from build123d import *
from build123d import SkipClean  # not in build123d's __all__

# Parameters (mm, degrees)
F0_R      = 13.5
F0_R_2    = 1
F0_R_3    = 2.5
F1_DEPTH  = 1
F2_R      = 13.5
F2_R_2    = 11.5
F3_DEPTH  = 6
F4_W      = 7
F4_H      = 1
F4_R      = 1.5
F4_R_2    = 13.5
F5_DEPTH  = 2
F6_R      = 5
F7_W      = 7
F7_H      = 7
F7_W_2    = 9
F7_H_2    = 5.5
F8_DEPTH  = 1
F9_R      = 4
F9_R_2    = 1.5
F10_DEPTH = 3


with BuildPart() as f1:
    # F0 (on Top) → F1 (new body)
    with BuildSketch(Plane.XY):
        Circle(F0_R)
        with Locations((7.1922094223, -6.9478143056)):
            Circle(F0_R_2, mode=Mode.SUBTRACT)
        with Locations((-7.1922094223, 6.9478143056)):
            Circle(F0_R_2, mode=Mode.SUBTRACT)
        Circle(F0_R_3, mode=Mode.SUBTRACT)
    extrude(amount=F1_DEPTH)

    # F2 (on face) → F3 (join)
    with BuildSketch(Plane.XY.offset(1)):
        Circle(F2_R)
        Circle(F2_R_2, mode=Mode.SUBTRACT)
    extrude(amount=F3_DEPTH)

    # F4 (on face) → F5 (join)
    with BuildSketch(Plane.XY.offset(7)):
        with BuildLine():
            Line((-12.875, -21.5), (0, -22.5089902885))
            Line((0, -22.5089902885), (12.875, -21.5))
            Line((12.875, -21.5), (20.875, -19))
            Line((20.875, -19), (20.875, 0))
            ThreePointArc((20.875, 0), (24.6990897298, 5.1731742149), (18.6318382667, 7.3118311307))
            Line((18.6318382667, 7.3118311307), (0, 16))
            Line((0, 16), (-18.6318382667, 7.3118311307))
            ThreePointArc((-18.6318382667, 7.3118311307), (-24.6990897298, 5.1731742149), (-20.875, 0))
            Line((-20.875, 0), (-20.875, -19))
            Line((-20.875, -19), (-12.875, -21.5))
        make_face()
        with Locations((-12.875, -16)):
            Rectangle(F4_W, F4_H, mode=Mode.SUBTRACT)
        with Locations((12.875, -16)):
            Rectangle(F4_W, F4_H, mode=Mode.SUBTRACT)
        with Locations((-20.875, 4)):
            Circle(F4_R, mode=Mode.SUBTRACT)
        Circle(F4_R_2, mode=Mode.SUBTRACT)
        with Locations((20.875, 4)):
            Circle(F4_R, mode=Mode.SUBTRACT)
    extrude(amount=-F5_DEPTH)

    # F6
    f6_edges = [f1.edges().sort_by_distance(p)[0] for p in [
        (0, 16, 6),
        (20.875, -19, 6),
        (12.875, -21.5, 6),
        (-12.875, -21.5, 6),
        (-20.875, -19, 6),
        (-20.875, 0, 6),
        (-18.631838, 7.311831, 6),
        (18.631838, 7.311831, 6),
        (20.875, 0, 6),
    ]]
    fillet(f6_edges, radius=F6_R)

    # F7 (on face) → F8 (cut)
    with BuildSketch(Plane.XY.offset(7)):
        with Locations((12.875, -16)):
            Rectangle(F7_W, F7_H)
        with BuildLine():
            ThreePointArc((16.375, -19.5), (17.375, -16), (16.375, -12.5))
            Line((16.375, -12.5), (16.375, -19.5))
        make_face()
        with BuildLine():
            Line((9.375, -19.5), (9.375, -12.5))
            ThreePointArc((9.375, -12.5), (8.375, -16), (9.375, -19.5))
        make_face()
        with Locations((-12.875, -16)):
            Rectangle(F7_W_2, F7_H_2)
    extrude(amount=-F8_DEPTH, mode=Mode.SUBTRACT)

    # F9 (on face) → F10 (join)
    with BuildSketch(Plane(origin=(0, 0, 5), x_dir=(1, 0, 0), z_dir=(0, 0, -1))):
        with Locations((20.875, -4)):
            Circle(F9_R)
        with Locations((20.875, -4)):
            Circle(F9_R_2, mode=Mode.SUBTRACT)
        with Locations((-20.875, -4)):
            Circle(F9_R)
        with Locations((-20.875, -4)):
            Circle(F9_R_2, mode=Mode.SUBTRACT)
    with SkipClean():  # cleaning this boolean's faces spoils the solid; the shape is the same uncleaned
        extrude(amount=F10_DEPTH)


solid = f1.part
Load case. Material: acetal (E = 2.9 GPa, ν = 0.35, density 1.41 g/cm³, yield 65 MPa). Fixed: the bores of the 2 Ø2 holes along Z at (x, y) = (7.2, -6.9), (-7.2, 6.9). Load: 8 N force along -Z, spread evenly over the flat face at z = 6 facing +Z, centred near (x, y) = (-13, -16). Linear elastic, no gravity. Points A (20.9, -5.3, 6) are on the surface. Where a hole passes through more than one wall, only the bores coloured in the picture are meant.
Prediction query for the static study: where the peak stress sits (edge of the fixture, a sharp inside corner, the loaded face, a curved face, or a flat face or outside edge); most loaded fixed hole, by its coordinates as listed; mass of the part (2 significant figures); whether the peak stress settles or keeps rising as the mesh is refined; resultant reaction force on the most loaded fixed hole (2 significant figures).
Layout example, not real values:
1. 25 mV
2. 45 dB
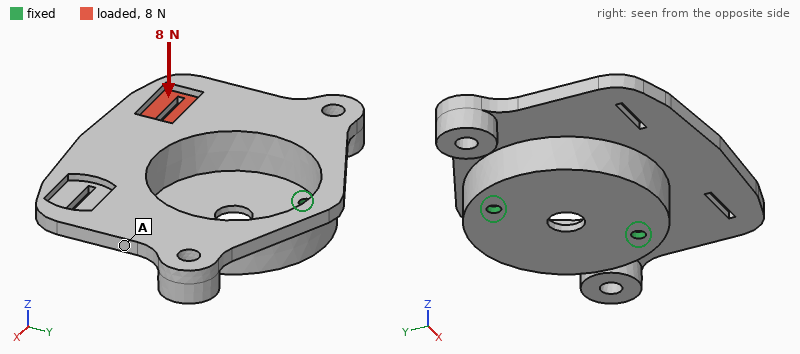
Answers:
1. edge of the fixture
2. (7.2, -6.9)
3. 4.6 g
4. keeps rising
5. 4.7 N
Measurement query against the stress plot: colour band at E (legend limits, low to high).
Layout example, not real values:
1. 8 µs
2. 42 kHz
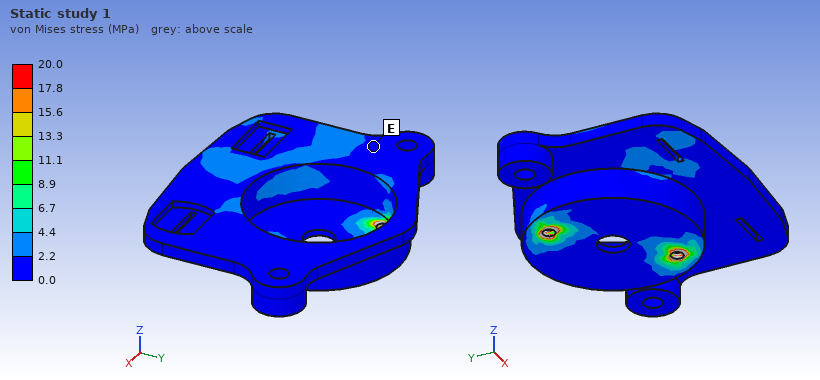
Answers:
1. 0.0 to 2.2 MPa
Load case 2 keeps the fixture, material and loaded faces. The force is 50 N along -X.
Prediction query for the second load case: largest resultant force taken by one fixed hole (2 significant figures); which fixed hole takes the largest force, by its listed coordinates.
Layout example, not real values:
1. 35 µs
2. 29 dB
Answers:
1. 60 N
2. (7.2, -6.9)
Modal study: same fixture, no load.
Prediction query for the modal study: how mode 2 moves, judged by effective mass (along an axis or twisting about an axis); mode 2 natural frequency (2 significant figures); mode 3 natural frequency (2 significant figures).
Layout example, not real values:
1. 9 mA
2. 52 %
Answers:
1. along Z
2. 1800 Hz
3. 2000 Hz
